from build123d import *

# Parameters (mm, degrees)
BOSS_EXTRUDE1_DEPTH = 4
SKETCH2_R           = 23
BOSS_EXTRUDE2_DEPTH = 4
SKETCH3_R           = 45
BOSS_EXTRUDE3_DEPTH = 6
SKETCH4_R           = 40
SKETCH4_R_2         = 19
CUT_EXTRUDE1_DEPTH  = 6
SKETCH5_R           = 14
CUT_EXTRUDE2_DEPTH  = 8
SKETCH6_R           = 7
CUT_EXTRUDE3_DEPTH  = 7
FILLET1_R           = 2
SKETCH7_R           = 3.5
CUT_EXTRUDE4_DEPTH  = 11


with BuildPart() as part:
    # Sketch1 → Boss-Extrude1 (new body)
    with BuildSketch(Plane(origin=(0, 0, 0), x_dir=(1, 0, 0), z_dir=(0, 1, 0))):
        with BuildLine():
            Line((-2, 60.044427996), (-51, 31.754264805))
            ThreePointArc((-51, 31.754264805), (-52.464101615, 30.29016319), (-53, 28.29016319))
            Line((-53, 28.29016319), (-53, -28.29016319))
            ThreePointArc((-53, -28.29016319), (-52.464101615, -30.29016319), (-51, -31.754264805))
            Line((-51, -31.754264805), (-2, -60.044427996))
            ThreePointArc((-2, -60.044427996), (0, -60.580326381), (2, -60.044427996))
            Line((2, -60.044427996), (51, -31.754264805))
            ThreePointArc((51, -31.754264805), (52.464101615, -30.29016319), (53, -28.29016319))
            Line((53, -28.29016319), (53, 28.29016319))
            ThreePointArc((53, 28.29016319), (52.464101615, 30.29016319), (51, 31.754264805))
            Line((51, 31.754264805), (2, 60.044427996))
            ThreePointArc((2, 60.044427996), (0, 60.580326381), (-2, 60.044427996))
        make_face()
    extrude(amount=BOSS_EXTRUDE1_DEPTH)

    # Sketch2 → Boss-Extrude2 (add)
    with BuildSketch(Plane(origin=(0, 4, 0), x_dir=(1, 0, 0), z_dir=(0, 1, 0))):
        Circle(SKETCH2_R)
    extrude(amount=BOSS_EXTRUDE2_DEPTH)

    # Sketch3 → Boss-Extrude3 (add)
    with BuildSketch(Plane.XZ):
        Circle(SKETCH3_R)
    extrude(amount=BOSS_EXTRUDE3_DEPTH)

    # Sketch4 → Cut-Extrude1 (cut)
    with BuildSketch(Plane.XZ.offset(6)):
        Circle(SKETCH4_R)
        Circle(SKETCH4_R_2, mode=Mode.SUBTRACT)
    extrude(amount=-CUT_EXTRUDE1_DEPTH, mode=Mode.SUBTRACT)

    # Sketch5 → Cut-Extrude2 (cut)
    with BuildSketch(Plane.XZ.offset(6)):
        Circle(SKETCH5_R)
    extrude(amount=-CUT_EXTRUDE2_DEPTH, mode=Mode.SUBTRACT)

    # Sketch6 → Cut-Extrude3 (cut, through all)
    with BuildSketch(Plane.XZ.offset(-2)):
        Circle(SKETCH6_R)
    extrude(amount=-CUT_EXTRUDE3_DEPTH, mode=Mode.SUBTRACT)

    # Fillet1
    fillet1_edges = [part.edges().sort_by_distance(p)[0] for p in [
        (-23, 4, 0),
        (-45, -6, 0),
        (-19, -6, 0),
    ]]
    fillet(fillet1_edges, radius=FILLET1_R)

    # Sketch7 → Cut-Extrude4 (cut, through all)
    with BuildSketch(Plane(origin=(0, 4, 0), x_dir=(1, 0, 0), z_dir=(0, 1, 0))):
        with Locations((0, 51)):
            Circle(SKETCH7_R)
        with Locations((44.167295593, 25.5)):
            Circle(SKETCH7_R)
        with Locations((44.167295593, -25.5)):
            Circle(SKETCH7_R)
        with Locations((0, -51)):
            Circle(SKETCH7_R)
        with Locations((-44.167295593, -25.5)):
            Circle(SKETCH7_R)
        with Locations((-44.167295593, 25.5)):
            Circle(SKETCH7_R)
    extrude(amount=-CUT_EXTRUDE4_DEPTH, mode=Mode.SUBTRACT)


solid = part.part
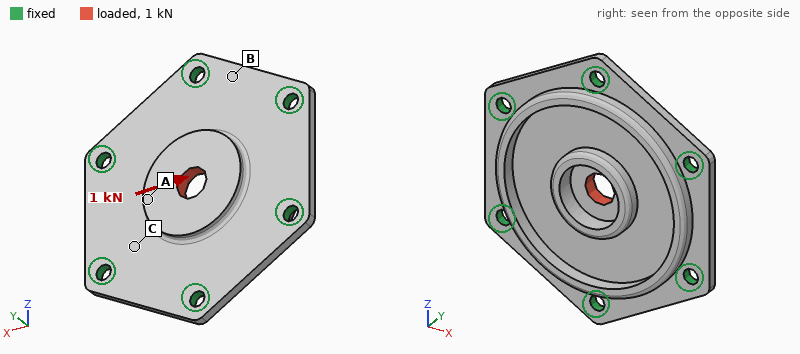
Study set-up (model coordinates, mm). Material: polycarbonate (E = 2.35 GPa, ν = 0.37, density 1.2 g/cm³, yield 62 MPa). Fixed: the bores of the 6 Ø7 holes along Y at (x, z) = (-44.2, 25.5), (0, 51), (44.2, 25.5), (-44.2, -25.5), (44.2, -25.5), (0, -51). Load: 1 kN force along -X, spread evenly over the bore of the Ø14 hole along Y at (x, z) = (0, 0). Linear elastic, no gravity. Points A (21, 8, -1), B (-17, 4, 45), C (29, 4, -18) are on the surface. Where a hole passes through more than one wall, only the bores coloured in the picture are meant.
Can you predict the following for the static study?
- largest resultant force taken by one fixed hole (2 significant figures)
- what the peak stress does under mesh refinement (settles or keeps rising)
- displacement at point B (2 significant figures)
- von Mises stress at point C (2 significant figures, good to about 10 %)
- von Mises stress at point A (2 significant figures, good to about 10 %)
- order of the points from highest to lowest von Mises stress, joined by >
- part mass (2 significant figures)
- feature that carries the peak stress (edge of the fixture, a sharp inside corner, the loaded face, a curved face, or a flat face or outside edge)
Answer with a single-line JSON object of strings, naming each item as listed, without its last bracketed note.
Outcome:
{"largest resultant force taken by one fixed hole": "220 N", "what the peak stress does under mesh refinement": "keeps rising", "displacement at point B": "11 µm", "von Mises stress at point C": "2.9 MPa", "von Mises stress at point A": "1.6 MPa", "order of the points from highest to lowest von Mises stress, joined by >": "C > A > B", "part mass": "64 g", "feature that carries the peak stress": "edge of the fixture"}
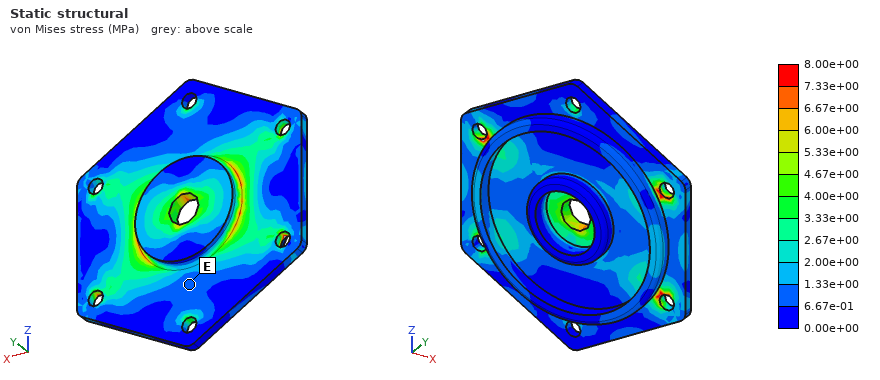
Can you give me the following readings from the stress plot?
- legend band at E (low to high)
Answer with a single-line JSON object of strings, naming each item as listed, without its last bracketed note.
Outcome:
{"legend band at E": "6.67e-01 to 1.33e+00 MPa"}
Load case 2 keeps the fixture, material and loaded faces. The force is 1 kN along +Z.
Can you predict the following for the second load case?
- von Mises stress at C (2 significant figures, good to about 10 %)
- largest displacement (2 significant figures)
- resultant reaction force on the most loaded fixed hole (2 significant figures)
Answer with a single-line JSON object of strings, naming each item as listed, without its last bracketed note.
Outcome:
{"von Mises stress at C": "1.8 MPa", "largest displacement": "68 µm", "resultant reaction force on the most loaded fixed hole": "250 N"}
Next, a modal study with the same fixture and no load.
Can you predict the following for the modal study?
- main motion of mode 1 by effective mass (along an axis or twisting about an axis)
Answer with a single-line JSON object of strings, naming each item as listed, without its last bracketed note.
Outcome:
{"main motion of mode 1 by effective mass": "along Y"}
